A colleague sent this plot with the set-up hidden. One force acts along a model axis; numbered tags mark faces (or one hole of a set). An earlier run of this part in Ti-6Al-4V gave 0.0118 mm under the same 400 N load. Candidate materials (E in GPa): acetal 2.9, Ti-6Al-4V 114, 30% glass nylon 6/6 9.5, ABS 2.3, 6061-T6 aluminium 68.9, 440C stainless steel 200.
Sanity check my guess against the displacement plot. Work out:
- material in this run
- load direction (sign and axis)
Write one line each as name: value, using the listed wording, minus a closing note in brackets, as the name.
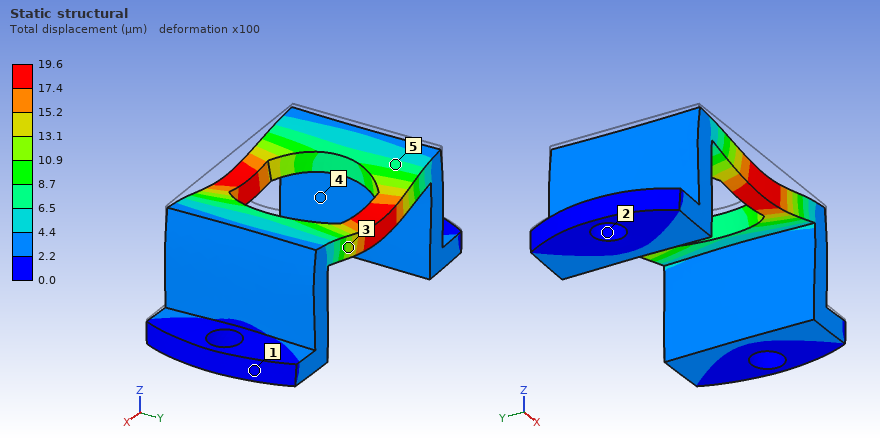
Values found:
material in this run: 6061-T6 aluminium
load direction: -Z
